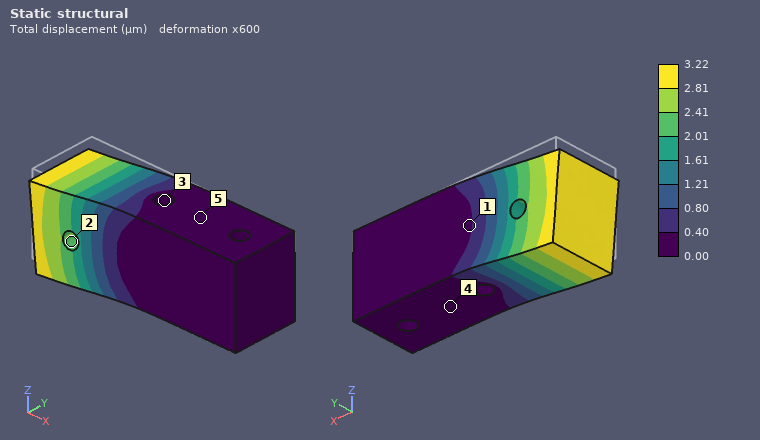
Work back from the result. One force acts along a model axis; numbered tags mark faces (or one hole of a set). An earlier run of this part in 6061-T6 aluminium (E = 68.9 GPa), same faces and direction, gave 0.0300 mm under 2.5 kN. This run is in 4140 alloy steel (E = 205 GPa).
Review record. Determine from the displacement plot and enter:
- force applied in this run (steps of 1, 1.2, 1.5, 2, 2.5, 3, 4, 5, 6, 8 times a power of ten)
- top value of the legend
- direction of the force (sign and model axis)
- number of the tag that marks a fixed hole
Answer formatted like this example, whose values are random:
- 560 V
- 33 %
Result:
- 800 N
- 3.22 µm
- -Z
- 3
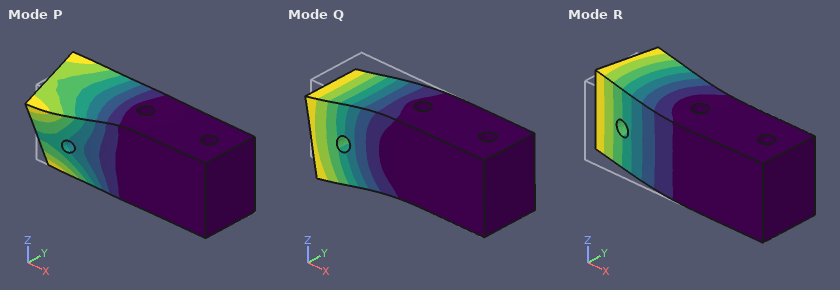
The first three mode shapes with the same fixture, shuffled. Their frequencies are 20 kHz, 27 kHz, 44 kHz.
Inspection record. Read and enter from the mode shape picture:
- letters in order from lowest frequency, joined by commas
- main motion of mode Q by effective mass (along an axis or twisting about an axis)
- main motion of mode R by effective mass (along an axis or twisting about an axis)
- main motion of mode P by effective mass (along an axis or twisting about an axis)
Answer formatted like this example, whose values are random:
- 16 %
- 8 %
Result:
- R, Q, P
- along Z
- along Y
- twisting about X
